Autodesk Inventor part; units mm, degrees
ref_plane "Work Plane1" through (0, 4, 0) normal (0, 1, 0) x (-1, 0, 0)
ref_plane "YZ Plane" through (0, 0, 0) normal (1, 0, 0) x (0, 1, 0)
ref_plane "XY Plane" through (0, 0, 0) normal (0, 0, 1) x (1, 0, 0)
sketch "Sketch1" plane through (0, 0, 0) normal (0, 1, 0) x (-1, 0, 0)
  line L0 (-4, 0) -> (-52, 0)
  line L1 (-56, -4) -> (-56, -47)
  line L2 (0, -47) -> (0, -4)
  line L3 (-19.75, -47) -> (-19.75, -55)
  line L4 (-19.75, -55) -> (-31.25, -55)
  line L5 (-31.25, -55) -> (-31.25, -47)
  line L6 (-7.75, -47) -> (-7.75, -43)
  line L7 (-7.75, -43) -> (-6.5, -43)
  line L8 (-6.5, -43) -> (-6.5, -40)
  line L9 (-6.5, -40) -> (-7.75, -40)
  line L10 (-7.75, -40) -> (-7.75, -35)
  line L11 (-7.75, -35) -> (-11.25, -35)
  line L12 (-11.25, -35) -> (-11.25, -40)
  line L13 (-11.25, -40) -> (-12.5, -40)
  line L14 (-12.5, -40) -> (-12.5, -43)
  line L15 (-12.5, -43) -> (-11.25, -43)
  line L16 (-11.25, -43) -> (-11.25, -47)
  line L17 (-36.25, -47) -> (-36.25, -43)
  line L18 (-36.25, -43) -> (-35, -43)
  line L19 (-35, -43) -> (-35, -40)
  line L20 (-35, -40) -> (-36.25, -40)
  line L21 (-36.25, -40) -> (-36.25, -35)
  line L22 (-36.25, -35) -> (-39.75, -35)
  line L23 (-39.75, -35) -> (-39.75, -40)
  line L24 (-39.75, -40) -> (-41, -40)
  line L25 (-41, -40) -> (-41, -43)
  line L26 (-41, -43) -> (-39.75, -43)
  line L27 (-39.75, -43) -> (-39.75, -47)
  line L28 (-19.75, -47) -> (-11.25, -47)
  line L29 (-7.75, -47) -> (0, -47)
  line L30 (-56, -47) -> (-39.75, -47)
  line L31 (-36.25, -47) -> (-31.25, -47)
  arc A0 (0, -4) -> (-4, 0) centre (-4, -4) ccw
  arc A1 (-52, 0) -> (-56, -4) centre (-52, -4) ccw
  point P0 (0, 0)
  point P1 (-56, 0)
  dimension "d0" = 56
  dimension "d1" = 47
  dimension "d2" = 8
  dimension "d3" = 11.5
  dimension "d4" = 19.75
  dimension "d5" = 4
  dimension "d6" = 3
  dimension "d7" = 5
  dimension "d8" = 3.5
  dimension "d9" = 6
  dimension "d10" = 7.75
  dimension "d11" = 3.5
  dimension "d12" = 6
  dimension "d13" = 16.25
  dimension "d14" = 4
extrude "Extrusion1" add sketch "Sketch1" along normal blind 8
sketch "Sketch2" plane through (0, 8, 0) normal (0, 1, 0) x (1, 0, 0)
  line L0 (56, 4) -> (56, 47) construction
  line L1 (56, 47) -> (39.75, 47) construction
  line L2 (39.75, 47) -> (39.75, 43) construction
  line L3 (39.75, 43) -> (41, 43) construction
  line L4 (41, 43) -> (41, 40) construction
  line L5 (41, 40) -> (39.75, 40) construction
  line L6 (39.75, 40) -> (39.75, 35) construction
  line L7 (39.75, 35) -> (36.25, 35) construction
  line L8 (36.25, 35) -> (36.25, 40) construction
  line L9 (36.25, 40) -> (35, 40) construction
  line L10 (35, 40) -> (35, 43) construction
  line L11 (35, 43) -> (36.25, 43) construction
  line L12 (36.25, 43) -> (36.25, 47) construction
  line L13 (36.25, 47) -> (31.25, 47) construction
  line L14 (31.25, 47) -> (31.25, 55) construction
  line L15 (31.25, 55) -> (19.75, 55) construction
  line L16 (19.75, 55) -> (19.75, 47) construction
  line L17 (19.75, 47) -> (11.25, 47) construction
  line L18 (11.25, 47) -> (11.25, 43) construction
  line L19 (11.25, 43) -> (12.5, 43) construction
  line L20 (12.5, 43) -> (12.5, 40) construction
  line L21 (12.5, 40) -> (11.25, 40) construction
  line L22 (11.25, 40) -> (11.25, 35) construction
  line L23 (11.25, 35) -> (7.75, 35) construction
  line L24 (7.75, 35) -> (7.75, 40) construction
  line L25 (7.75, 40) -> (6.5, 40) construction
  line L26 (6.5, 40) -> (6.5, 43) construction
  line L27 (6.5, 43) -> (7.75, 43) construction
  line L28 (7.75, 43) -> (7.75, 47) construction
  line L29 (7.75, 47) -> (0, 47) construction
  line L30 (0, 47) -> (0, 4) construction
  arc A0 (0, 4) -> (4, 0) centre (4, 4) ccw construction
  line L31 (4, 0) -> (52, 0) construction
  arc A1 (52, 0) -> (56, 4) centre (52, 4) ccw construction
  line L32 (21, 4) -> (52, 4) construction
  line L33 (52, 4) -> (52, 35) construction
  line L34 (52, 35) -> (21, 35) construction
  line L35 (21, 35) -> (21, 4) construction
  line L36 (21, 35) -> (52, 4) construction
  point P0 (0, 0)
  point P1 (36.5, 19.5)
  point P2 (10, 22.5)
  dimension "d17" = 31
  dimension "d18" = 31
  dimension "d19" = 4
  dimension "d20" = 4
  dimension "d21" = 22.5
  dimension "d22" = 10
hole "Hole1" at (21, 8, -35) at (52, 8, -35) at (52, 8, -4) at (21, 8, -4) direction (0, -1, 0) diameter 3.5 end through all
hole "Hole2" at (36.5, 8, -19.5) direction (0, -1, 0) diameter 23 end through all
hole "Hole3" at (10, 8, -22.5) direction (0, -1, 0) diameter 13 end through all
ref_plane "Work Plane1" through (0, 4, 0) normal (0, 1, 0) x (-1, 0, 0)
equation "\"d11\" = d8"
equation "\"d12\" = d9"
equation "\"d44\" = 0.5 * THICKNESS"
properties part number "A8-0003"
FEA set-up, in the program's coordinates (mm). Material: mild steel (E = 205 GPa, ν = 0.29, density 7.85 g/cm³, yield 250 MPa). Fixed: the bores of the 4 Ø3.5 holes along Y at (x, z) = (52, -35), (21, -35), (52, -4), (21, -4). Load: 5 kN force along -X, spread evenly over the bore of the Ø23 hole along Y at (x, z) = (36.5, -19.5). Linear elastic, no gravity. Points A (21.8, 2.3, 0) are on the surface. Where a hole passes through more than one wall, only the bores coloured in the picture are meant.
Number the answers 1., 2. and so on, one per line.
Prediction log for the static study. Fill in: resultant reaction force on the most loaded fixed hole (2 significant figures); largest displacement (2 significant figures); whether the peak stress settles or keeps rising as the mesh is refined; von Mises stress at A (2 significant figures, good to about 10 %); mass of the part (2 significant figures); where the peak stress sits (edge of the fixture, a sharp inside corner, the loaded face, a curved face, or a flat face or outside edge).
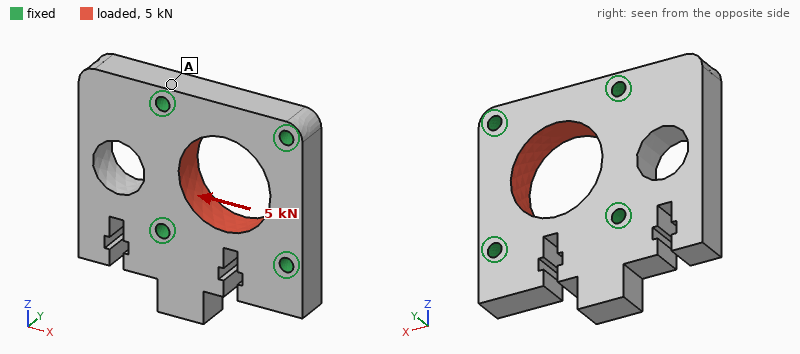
1. 1.4 kN
2. 2.6 µm
3. keeps rising
4. 7.2 MPa
5. 130 g
6. edge of the fixture
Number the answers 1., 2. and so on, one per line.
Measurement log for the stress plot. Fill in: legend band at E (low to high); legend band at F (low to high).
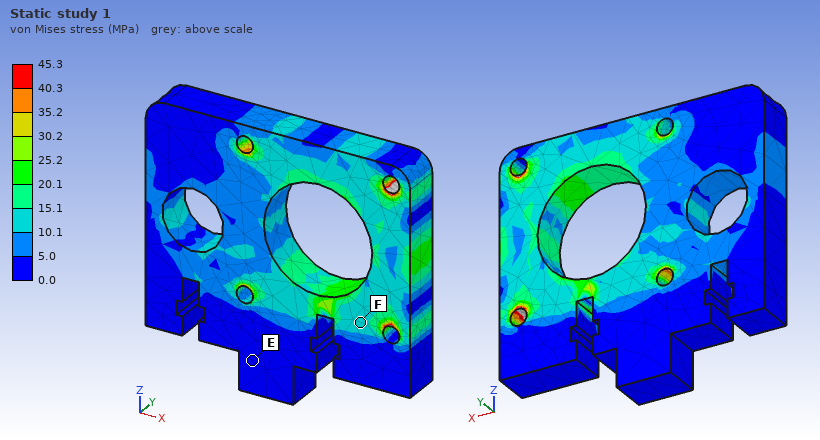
1. 0.0 to 5.0 MPa
2. 10.1 to 15.1 MPa
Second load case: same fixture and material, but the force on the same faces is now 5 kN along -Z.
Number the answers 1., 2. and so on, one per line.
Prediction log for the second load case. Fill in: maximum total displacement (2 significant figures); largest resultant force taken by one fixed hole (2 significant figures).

1. 2.7 µm
2. 1.5 kN
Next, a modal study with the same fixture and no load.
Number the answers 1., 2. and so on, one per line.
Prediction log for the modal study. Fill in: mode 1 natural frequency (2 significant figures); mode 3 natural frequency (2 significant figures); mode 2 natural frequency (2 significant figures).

1. 9400 Hz
2. 15 kHz
3. 13 kHz
